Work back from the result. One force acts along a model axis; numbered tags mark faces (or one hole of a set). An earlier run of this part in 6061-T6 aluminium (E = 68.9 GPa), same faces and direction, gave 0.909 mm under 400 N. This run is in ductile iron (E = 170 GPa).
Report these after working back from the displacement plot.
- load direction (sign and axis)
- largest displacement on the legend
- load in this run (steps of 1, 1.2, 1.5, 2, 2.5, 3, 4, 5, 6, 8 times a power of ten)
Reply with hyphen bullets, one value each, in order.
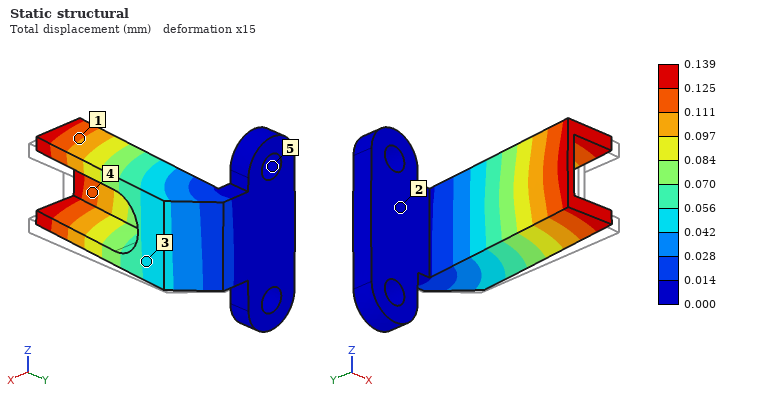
- -X
- 0.139 mm
- 150 N
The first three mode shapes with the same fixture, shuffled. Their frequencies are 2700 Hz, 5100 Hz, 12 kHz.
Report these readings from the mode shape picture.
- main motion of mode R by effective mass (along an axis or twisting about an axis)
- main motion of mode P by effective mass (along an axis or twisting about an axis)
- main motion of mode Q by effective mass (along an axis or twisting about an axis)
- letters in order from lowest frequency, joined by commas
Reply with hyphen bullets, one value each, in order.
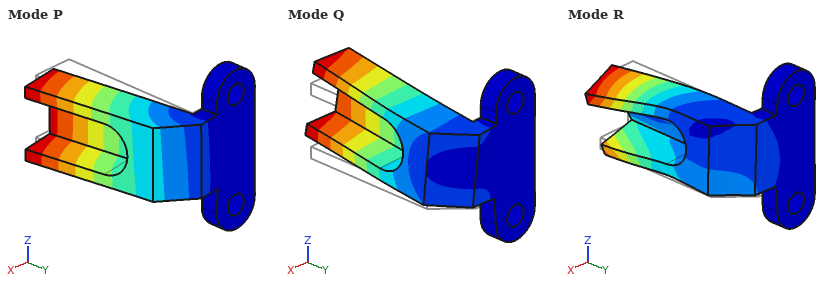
- along Y
- along X
- along Z
- P, Q, R
